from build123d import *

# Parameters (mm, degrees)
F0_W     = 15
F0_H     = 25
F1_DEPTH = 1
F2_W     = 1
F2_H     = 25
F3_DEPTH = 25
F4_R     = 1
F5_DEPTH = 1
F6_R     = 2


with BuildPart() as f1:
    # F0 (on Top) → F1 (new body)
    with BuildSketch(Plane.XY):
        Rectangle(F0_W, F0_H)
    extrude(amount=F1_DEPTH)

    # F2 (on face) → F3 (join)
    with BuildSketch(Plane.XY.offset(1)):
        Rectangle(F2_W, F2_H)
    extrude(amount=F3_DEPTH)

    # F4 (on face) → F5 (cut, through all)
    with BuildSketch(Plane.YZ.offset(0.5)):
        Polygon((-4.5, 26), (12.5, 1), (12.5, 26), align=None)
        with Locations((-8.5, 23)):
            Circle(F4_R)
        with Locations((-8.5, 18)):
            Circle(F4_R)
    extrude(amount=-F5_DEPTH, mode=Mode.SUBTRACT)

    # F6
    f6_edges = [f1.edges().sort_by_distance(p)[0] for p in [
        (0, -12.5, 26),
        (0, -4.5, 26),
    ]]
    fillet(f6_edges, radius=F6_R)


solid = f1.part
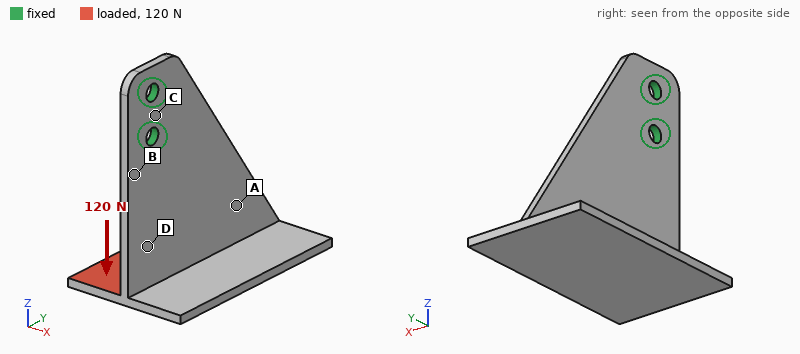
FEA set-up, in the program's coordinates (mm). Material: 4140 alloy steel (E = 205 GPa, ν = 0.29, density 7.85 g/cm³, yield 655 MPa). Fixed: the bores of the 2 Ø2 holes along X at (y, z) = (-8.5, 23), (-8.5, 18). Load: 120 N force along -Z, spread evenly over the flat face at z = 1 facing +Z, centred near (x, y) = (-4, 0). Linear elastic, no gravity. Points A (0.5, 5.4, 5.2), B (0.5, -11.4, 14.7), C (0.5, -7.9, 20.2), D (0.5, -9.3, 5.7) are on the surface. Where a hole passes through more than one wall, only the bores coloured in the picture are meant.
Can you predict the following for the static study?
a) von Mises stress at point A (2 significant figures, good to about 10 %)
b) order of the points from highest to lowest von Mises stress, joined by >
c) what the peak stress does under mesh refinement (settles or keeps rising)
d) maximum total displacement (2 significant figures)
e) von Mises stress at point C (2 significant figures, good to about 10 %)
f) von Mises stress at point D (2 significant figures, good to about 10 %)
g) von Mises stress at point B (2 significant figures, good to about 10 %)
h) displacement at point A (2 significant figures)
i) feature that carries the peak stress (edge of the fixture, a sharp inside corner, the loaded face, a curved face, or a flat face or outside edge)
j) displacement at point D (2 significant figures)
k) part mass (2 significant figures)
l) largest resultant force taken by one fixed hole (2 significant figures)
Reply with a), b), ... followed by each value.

a) 110 MPa
b) B > D > A > C
c) keeps rising
d) 0.43 mm
e) 53 MPa
f) 140 MPa
g) 230 MPa
h) 0.19 mm
i) edge of the fixture
j) 0.14 mm
k) 6.1 g
l) 160 N
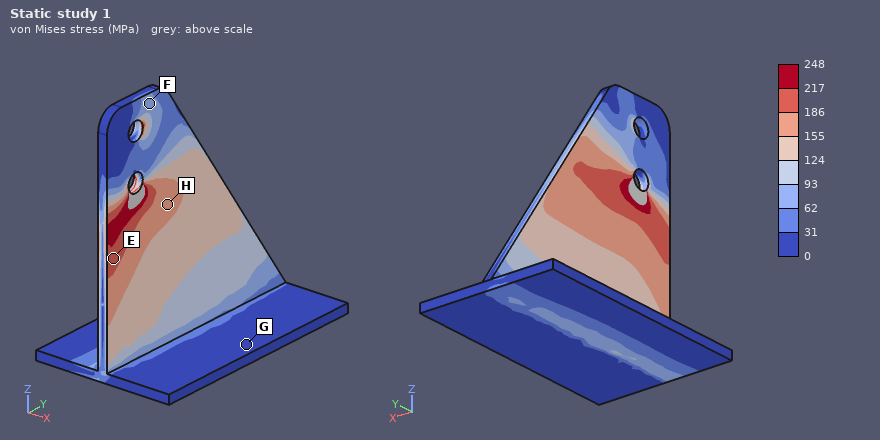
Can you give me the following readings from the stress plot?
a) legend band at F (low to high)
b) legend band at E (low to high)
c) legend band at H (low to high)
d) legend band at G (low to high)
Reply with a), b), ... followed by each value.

a) 62 to 93 MPa
b) 186 to 217 MPa
c) 155 to 186 MPa
d) 0 to 31 MPa
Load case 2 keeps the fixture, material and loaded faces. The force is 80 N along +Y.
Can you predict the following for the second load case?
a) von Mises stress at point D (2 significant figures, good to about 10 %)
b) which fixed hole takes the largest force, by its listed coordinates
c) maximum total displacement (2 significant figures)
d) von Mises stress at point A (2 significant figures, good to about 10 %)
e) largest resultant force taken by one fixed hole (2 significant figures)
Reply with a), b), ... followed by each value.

a) 84 MPa
b) (-8.5, 18)
c) 0.27 mm
d) 29 MPa
e) 260 N
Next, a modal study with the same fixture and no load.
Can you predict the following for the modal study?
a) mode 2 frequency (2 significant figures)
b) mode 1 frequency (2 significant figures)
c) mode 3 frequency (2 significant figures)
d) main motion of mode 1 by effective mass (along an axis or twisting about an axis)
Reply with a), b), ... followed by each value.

a) 1800 Hz
b) 800 Hz
c) 4800 Hz
d) along X
